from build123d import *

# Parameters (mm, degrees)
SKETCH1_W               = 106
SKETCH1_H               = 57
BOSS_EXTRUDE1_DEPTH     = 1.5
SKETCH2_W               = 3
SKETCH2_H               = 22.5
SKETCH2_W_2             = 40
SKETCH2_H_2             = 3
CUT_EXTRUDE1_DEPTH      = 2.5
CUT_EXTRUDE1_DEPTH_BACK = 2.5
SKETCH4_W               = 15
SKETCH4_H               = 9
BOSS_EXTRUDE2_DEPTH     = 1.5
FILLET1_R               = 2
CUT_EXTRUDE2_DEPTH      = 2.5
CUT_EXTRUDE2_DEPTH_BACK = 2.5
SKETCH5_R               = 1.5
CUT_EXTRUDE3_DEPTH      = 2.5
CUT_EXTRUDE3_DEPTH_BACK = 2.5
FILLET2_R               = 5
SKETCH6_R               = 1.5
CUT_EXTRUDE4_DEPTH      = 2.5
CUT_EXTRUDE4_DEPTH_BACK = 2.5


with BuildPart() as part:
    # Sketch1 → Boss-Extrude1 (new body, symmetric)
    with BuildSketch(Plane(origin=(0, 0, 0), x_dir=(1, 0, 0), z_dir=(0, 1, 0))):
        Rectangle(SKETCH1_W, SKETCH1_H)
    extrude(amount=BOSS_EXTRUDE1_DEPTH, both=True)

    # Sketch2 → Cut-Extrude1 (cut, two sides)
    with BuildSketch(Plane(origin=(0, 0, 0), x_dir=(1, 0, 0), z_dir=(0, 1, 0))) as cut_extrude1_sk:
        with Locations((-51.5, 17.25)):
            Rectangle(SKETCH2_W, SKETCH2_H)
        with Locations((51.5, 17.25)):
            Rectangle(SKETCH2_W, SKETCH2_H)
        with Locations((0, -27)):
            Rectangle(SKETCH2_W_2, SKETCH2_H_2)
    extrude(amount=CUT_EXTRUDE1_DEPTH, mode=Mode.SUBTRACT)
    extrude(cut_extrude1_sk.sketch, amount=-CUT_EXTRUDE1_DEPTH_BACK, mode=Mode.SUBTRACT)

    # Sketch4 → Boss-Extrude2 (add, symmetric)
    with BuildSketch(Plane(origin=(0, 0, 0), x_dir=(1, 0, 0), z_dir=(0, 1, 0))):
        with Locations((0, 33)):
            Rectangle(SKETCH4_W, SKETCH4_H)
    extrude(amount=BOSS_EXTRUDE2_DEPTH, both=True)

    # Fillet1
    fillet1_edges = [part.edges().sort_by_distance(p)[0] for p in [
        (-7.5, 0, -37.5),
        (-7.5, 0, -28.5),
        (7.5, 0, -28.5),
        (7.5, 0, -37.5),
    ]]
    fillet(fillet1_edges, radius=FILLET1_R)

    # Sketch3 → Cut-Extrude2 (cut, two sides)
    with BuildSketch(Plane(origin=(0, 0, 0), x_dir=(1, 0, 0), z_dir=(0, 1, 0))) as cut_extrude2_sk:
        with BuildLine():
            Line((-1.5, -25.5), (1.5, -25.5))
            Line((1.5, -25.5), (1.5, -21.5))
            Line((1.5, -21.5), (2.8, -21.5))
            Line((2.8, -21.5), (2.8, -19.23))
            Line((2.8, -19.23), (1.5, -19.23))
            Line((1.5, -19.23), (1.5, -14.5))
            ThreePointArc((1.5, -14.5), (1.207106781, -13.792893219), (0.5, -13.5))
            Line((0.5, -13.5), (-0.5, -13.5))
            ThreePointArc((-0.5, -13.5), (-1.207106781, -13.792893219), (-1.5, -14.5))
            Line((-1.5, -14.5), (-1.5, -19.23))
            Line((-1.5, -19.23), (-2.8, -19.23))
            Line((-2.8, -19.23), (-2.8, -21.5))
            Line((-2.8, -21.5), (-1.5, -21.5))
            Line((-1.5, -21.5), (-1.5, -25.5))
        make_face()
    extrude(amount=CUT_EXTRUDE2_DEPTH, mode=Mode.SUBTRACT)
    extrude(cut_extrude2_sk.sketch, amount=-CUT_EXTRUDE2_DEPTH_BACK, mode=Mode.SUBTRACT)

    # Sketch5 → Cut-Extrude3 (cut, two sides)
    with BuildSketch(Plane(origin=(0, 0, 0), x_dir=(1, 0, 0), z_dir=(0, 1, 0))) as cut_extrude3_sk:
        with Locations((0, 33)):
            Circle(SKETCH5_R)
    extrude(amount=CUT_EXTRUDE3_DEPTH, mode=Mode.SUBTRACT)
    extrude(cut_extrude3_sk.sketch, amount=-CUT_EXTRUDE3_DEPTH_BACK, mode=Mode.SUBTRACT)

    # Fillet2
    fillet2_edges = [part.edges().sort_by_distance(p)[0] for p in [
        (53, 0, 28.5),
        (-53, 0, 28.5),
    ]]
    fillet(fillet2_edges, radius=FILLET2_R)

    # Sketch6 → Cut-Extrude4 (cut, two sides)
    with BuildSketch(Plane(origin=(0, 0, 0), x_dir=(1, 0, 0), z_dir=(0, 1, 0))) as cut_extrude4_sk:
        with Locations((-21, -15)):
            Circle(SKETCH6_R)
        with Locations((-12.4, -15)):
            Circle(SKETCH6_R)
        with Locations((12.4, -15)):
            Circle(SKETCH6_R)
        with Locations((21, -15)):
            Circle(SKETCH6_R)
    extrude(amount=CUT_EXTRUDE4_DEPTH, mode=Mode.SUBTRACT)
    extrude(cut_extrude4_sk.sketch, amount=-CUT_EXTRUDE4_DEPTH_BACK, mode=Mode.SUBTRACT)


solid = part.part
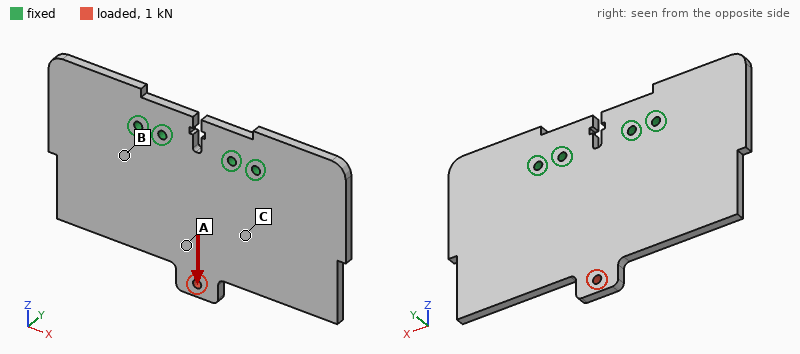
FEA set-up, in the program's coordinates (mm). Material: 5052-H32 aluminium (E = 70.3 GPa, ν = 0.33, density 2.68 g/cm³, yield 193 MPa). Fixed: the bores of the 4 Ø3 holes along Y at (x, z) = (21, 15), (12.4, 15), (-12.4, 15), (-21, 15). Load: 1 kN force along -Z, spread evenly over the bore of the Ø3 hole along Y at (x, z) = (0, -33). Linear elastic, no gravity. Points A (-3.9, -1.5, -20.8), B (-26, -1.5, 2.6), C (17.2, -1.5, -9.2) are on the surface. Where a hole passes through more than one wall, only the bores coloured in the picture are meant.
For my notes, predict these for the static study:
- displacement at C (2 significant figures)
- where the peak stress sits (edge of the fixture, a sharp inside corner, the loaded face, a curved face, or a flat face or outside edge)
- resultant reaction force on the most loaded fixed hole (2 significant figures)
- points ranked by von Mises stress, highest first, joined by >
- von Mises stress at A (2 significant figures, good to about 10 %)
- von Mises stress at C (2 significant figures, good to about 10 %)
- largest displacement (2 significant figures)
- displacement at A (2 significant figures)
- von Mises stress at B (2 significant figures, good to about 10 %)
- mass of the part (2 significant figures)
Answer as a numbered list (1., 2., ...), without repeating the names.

1. 2.2 µm
2. the loaded face
3. 270 N
4. A > C > B
5. 15 MPa
6. 5.9 MPa
7. 11 µm
8. 4.9 µm
9. 3.3 MPa
10. 47 g
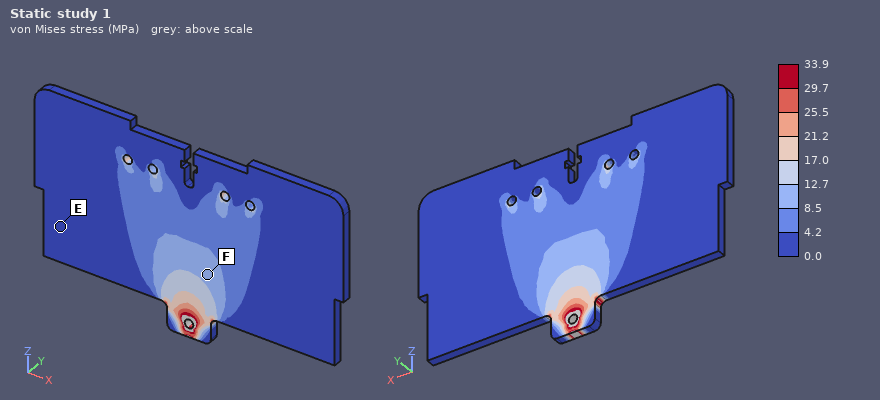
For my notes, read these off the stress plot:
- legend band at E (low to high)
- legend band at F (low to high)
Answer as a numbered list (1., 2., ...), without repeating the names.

1. 0.0 to 4.2 MPa
2. 8.5 to 12.7 MPa
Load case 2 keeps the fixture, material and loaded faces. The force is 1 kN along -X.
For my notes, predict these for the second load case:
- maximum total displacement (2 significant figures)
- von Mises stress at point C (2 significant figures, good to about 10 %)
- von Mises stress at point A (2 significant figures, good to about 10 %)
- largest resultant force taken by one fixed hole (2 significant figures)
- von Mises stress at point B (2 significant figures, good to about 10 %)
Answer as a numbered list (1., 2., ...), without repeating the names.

1. 36 µm
2. 14 MPa
3. 10 MPa
4. 1.0 kN
5. 11 MPa
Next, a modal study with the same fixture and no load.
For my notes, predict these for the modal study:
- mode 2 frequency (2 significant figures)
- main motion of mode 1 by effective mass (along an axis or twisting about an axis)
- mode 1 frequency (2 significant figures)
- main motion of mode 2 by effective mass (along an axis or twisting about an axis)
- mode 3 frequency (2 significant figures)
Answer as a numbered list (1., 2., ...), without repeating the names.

1. 1400 Hz
2. along Y
3. 1100 Hz
4. twisting about Z
5. 2000 Hz
